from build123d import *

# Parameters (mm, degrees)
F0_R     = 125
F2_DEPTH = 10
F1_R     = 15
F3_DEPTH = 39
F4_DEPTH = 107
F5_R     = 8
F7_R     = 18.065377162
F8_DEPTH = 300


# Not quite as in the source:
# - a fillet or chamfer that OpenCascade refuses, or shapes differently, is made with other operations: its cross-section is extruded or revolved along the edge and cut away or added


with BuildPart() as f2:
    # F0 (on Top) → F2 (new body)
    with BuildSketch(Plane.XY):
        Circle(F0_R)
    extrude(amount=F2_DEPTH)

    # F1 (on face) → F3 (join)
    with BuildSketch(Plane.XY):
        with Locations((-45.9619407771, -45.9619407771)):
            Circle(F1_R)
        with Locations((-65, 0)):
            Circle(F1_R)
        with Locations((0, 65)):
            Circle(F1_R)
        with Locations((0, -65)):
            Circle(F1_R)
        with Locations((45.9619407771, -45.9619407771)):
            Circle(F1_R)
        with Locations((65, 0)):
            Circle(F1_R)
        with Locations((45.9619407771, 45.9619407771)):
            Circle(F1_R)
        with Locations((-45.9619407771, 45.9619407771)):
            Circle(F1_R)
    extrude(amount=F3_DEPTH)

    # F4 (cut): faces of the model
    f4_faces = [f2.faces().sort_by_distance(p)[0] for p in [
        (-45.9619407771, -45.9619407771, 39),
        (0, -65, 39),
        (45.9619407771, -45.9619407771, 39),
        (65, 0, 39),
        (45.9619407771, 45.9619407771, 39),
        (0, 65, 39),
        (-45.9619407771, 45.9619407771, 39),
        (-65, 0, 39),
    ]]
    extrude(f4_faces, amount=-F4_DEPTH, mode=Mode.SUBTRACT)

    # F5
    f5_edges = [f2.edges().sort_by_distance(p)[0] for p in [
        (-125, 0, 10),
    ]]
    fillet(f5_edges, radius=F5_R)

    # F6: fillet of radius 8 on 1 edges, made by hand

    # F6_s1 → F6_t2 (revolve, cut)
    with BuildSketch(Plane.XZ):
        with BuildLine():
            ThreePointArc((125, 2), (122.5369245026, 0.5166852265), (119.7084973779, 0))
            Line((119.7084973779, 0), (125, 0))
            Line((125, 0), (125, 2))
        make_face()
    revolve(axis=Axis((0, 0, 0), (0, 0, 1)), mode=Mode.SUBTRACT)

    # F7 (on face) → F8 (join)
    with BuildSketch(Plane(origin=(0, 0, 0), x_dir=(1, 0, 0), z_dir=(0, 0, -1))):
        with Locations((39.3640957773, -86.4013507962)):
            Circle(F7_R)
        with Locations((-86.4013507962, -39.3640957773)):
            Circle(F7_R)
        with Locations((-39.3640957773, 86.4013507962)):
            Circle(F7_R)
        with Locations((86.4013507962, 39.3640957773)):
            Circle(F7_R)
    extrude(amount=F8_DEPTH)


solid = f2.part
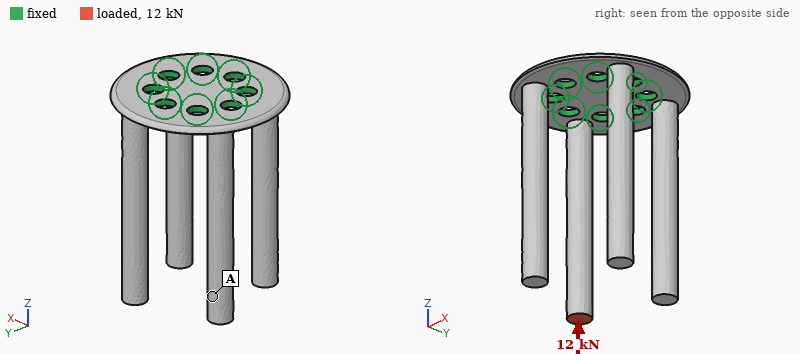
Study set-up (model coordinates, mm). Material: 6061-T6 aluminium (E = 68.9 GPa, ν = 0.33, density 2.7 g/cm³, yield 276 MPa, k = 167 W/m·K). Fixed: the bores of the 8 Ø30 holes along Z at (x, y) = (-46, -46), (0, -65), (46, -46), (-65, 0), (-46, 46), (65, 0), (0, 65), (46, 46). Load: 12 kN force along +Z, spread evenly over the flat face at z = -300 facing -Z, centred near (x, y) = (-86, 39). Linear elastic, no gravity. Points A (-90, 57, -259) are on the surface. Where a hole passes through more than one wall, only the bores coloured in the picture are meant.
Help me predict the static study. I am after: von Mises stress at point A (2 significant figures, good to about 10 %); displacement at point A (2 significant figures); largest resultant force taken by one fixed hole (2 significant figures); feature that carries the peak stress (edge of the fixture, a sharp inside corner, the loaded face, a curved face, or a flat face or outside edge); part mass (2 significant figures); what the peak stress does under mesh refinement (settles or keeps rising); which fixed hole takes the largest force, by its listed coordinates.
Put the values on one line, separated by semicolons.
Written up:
12 MPa; 1.2 mm; 7.1 kN; edge of the fixture; 4.5 kg; keeps rising; (-46, 46)
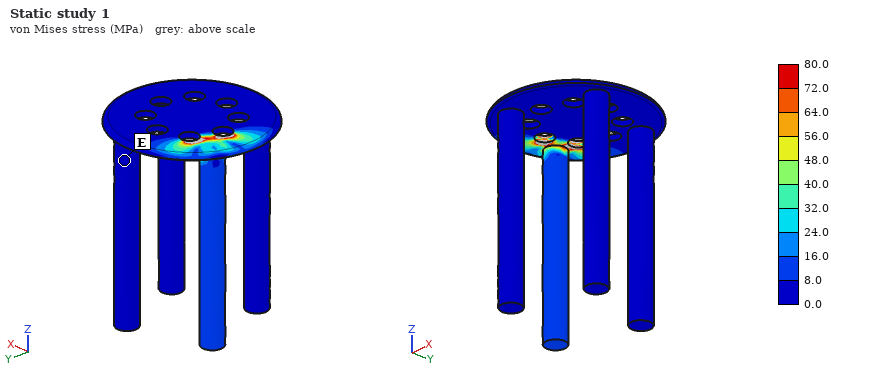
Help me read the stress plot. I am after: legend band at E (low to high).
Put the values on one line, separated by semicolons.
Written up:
0.0 to 8.0 MPa
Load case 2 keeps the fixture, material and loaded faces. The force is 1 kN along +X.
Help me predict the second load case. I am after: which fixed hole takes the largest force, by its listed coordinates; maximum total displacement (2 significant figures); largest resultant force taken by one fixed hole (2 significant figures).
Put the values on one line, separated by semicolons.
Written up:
(-65, 0); 3.6 mm; 3.7 kN
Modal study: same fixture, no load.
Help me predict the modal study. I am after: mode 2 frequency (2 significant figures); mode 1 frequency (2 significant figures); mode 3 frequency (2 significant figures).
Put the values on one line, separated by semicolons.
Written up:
160 Hz; 160 Hz; 160 Hz
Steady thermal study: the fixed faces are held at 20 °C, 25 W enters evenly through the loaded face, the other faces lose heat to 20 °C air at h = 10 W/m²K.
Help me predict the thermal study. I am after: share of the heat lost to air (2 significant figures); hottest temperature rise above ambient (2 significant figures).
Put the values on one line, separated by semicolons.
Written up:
28 %; 39 K
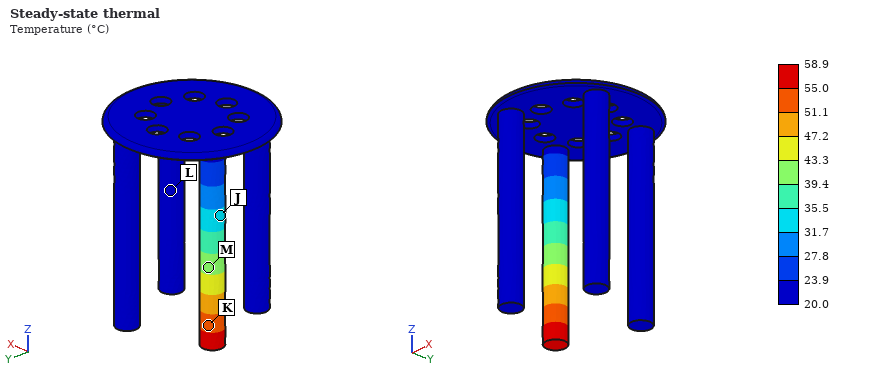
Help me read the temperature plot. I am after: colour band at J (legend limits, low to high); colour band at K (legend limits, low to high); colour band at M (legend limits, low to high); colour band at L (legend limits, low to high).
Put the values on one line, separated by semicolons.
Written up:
31.7 to 35.5 °C; 51.1 to 55.0 °C; 39.4 to 43.3 °C; 20.0 to 23.9 °C
